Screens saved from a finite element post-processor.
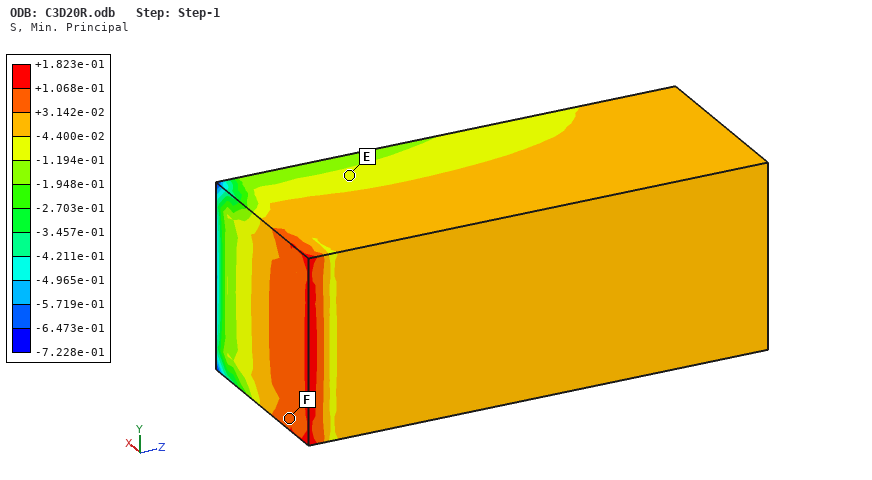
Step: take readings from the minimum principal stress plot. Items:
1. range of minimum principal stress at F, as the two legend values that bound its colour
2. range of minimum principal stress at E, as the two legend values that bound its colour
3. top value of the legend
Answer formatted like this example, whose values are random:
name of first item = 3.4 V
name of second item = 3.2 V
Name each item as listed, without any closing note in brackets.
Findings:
range of minimum principal stress at F, as the two legend values that bound its colour = +3.142e-02 to +1.068e-01
range of minimum principal stress at E, as the two legend values that bound its colour = -1.194e-01 to -4.400e-02
top value of the legend = +1.823e-01
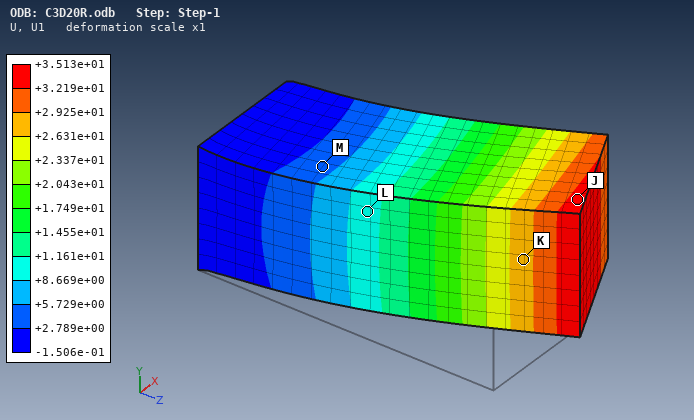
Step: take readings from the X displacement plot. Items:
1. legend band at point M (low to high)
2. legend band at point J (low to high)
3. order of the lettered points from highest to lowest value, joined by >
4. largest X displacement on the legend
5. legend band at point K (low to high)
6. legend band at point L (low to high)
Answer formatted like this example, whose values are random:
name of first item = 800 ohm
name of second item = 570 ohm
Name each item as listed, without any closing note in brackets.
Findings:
legend band at point M = +2.789e+00 to +5.729e+00
legend band at point J = +3.219e+01 to +3.513e+01
order of the lettered points from highest to lowest value, joined by > = J > K > L > M
largest X displacement on the legend = +3.513e+01
legend band at point K = +2.631e+01 to +2.925e+01
legend band at point L = +8.669e+00 to +1.161e+01
